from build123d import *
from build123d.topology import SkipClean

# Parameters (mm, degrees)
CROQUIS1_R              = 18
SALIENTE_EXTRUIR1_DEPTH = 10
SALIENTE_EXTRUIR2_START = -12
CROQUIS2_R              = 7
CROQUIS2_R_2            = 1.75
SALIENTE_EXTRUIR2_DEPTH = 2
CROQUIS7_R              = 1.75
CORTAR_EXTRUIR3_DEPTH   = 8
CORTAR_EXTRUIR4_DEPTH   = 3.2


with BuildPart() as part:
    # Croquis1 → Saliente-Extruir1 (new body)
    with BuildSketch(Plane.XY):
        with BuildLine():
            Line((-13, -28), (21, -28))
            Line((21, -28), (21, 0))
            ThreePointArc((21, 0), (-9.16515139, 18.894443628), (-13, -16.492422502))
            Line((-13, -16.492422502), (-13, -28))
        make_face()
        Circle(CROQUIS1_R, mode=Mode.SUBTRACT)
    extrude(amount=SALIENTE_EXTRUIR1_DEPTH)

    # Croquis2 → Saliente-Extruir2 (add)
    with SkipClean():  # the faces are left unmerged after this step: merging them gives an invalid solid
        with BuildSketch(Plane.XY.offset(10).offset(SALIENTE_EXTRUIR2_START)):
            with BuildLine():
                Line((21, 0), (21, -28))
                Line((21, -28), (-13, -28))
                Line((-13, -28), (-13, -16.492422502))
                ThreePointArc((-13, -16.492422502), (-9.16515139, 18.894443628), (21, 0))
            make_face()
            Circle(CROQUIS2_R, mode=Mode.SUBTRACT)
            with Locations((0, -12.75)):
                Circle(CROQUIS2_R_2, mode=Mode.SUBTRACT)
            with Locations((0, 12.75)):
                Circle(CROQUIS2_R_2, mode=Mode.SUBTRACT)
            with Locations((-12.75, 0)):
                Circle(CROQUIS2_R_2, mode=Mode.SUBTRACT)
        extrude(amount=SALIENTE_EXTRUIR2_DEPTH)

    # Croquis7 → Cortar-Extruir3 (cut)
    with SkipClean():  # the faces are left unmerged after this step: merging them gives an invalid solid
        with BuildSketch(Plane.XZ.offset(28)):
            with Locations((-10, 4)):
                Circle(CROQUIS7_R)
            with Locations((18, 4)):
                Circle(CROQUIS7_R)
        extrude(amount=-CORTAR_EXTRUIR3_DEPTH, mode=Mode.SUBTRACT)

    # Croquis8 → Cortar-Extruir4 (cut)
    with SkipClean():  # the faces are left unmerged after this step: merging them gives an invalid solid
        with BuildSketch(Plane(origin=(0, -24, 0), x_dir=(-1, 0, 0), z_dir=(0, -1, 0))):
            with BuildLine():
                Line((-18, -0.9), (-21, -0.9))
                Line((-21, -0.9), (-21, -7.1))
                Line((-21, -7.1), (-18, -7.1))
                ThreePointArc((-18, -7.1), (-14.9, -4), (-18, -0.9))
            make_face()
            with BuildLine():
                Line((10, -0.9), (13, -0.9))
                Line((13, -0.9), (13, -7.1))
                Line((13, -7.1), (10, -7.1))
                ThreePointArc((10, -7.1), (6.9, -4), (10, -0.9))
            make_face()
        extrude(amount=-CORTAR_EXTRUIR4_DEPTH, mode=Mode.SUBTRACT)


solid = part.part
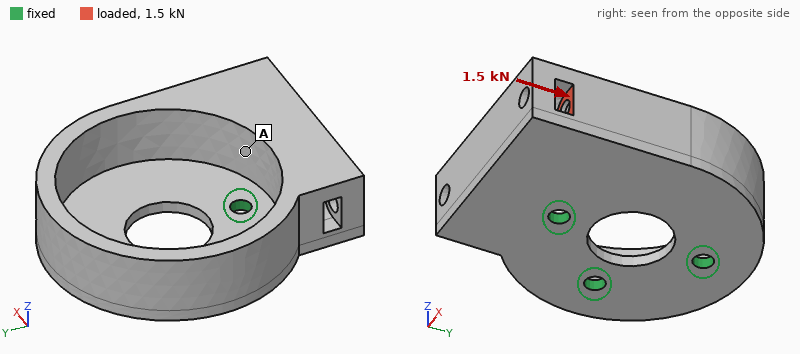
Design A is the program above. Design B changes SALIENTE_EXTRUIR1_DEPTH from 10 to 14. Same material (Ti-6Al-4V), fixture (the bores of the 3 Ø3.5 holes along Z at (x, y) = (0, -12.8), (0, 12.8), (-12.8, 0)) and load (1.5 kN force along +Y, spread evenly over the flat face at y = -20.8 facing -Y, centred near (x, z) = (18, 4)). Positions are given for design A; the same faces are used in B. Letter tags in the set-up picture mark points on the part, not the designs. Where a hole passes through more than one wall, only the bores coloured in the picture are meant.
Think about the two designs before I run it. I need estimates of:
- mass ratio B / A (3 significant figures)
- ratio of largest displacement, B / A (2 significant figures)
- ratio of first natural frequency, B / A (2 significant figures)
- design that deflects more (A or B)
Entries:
1.29
0.81
0.88
A
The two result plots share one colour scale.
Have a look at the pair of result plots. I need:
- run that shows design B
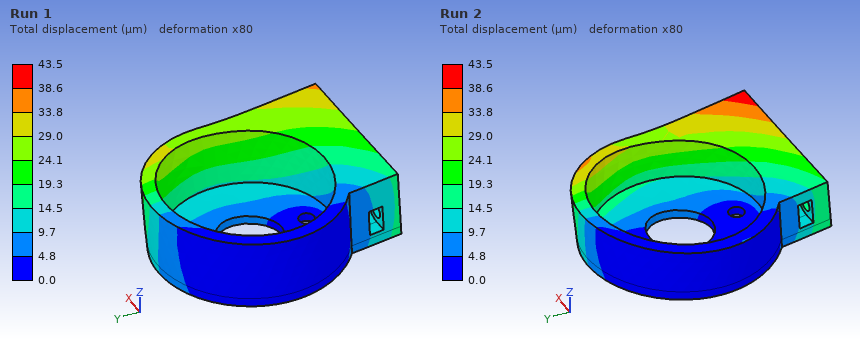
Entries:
Run 1
